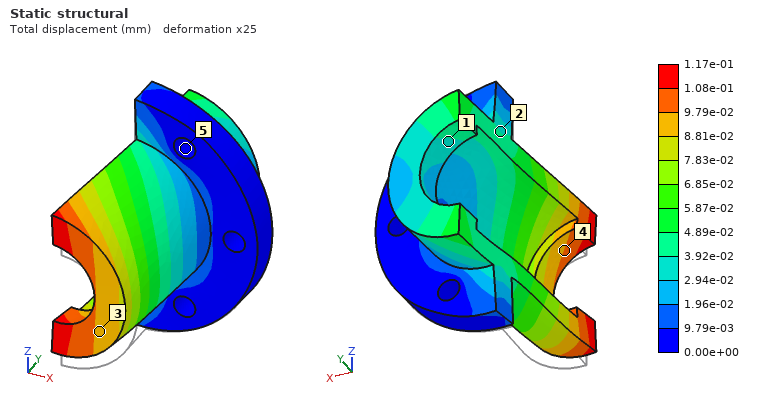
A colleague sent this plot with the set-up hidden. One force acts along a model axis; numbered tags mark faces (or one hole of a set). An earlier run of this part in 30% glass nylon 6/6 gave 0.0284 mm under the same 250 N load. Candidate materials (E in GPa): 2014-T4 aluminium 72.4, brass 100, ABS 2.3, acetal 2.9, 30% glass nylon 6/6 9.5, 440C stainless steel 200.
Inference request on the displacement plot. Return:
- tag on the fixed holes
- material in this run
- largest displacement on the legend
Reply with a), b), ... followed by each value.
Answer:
a) 5
b) ABS
c) 1.17e-01 mm
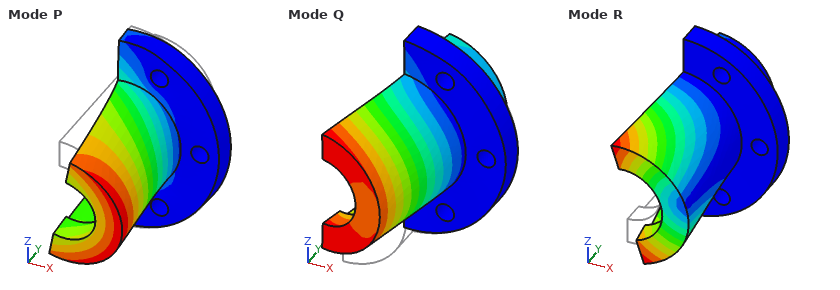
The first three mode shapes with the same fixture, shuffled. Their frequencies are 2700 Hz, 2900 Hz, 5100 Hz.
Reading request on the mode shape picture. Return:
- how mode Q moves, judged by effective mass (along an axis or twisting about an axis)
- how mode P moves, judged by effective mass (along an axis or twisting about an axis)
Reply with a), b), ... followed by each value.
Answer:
a) along X
b) along Z
